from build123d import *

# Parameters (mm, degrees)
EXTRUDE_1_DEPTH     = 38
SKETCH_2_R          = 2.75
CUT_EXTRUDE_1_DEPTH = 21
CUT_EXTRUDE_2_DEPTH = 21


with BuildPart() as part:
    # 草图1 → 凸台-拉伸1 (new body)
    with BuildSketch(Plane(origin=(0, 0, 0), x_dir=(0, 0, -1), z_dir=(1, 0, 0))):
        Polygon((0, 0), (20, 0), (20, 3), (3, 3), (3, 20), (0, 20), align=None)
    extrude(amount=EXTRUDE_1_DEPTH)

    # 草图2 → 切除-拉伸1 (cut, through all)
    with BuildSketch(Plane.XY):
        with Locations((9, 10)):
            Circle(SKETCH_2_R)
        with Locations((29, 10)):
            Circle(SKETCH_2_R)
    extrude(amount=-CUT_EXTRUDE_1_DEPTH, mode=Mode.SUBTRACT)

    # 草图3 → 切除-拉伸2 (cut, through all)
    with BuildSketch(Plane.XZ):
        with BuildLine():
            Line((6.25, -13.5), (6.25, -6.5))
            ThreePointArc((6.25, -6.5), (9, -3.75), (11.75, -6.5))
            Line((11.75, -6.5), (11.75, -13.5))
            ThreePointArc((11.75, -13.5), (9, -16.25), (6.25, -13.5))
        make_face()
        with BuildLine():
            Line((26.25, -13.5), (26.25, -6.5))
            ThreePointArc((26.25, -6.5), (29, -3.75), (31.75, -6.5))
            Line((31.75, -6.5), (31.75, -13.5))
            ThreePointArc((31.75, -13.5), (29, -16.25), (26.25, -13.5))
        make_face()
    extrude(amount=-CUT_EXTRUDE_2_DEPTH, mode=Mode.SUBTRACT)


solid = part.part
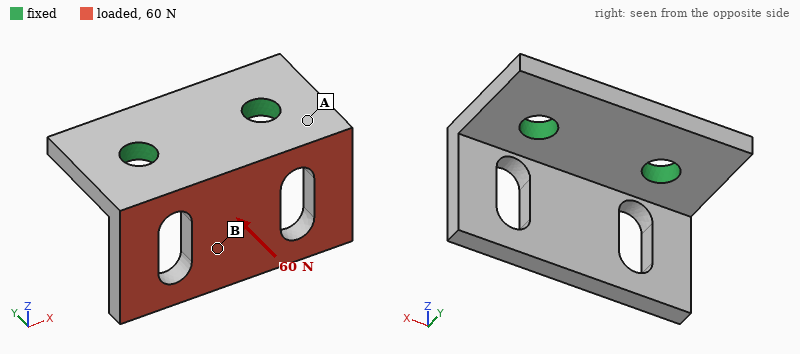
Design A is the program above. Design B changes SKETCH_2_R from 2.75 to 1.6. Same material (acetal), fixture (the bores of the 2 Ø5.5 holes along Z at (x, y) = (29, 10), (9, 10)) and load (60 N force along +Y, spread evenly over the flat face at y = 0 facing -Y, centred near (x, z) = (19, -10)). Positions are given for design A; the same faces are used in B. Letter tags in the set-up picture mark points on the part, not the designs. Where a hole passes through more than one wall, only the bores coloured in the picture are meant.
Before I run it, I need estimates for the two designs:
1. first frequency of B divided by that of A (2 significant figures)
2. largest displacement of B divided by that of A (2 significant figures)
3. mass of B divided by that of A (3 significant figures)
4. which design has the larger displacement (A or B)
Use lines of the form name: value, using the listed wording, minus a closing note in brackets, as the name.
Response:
first frequency of B divided by that of A: 0.92
largest displacement of B divided by that of A: 1.2
mass of B divided by that of A: 1.03
which design has the larger displacement: B
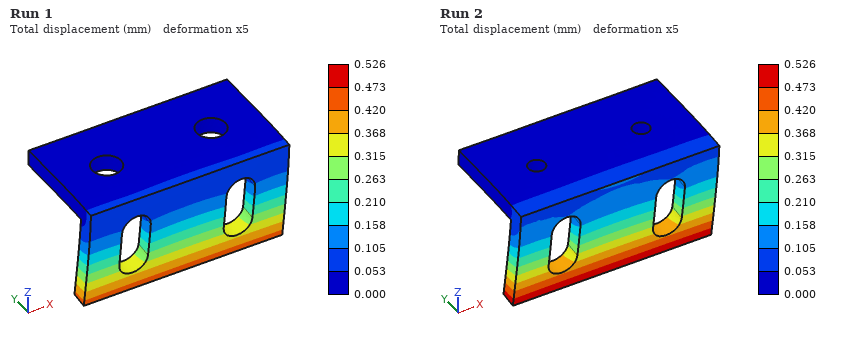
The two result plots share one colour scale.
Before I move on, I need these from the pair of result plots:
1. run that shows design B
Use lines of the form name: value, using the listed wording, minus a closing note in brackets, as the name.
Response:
run that shows design B: Run 2
